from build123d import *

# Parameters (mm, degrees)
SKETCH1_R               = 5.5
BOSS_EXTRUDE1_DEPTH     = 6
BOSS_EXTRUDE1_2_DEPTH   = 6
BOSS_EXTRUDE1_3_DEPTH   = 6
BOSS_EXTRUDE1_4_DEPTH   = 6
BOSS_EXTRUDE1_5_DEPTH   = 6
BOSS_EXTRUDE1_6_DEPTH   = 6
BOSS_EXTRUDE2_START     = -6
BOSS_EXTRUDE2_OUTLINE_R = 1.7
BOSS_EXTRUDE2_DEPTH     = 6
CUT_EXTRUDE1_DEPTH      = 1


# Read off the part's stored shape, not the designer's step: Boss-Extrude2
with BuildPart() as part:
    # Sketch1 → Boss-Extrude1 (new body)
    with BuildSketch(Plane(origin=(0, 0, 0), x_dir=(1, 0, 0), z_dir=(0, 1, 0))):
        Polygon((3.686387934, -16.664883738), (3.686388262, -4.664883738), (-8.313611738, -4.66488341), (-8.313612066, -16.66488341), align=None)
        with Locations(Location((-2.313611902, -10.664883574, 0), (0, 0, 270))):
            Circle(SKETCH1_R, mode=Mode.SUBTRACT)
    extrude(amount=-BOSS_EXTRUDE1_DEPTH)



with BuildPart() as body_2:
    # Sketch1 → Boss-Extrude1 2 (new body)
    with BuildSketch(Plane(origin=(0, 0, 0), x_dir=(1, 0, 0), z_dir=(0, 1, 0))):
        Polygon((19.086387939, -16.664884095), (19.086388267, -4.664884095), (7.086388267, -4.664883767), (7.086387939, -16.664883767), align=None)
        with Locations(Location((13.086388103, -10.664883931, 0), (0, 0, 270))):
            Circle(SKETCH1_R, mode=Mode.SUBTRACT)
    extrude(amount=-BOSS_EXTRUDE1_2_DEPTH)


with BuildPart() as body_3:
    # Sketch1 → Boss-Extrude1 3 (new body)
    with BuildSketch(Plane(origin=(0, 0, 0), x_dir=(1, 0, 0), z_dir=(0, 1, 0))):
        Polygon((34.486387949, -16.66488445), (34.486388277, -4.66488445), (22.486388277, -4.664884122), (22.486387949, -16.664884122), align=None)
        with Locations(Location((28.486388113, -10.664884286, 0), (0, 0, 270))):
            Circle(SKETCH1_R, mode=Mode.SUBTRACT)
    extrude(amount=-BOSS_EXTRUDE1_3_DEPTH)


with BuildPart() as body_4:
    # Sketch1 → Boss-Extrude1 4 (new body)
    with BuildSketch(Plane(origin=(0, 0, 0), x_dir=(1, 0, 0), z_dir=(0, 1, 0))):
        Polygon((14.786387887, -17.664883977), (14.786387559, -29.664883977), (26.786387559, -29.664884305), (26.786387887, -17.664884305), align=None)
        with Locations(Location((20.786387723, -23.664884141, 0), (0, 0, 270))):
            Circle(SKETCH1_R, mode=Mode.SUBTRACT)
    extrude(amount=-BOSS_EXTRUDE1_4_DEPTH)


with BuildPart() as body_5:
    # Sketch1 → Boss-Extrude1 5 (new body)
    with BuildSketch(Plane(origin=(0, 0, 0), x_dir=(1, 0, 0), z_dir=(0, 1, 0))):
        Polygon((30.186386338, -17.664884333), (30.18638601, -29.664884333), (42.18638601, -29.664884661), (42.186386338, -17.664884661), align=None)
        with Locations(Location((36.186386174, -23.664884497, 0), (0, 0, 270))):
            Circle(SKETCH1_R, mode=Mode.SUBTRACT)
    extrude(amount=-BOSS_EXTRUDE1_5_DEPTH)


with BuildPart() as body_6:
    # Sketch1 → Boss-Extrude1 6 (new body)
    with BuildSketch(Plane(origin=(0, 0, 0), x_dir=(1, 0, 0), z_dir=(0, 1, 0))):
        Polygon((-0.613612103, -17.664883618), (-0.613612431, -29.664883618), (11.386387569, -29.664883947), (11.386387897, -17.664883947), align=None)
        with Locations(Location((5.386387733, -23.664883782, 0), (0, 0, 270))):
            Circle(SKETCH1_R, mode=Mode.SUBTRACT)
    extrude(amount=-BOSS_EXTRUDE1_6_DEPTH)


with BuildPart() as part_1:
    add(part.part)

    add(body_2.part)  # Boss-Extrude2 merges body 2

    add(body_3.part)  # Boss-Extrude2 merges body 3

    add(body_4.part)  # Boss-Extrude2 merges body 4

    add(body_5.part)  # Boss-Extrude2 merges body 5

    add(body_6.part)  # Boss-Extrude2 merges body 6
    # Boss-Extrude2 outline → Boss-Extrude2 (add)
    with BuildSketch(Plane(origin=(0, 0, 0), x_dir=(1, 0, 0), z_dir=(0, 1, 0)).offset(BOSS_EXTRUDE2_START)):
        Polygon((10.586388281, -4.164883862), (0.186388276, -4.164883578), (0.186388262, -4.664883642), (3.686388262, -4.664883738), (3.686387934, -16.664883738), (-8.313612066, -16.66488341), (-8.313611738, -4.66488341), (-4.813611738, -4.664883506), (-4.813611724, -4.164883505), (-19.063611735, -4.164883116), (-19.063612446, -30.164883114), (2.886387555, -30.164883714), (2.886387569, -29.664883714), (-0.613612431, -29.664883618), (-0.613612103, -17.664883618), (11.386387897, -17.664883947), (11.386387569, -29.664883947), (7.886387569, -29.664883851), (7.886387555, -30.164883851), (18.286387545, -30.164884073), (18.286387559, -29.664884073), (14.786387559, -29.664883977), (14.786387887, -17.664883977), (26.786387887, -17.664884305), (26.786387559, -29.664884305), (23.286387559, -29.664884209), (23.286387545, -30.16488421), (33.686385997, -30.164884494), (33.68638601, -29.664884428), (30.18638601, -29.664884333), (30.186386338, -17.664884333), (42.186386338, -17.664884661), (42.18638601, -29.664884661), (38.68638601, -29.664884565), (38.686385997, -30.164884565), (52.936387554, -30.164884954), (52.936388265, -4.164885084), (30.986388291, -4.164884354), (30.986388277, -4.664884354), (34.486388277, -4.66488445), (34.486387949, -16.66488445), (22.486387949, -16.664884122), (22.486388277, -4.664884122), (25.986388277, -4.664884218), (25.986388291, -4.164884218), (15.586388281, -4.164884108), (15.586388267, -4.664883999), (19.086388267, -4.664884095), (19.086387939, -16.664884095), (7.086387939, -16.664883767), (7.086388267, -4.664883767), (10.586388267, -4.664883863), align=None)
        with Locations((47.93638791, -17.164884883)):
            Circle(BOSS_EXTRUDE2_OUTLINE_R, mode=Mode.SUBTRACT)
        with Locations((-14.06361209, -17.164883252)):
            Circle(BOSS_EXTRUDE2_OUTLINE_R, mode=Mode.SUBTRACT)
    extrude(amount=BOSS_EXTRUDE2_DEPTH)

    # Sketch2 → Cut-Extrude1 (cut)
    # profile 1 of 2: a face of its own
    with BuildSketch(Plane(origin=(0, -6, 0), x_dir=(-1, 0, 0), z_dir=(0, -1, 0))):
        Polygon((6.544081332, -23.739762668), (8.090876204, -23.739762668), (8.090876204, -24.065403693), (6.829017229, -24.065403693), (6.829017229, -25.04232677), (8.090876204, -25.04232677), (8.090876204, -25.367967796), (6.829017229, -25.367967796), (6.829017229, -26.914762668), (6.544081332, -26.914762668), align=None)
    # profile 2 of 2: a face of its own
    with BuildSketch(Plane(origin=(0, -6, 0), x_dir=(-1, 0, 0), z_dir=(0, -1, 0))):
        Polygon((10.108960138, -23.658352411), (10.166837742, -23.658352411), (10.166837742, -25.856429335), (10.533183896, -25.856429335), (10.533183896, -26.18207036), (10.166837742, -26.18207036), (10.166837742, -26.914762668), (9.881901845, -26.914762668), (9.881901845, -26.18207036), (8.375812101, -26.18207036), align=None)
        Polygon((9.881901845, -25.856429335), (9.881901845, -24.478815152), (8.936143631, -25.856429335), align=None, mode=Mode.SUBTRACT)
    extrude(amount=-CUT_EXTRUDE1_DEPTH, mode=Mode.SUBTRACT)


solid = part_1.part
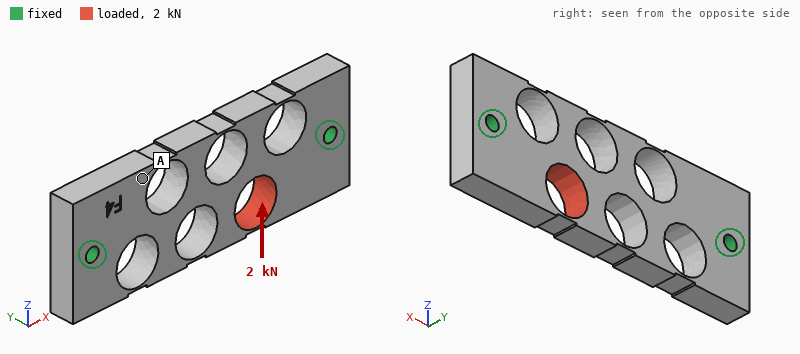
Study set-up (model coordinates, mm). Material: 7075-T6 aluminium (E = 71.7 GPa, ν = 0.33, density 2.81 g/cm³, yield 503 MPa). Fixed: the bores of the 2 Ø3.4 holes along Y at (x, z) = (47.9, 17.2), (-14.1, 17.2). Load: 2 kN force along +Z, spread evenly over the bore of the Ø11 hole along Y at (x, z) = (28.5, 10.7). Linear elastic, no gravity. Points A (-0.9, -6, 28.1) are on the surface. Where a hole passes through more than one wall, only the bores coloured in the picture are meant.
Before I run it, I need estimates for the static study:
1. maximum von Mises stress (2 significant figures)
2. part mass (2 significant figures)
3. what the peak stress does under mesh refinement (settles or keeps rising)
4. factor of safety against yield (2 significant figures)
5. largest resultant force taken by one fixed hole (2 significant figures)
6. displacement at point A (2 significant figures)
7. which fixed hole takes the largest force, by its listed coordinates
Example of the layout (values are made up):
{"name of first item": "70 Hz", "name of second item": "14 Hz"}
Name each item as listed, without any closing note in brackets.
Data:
{"maximum von Mises stress": "280 MPa", "part mass": "21 g", "what the peak stress does under mesh refinement": "settles", "factor of safety against yield": "1.8", "largest resultant force taken by one fixed hole": "1.5 kN", "displacement at point A": "20 µm", "which fixed hole takes the largest force, by its listed coordinates": "(47.9, 17.2)"}
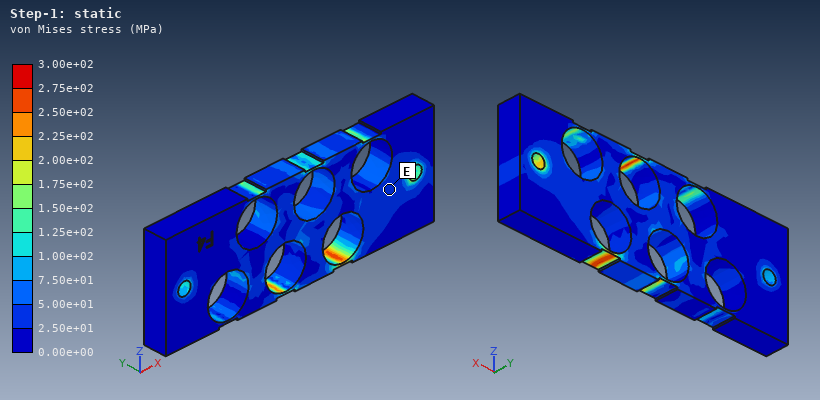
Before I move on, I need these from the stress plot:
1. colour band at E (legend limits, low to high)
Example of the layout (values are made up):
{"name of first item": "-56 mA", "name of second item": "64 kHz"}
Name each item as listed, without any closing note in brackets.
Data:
{"colour band at E": "2.50e+01 to 5.00e+01 MPa"}
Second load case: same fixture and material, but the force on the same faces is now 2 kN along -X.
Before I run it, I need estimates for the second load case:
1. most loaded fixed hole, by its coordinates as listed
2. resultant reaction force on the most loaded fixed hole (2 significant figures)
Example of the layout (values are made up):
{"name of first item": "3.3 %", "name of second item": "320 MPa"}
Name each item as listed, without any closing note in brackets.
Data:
{"most loaded fixed hole, by its coordinates as listed": "(47.9, 17.2)", "resultant reaction force on the most loaded fixed hole": "1.5 kN"}
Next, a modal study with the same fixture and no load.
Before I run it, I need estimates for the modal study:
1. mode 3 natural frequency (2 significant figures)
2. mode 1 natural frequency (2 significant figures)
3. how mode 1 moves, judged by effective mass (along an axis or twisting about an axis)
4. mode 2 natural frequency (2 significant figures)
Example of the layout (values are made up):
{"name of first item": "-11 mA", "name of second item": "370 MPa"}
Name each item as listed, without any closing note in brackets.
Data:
{"mode 3 natural frequency": "9900 Hz", "mode 1 natural frequency": "6700 Hz", "how mode 1 moves, judged by effective mass": "along Y", "mode 2 natural frequency": "9500 Hz"}
